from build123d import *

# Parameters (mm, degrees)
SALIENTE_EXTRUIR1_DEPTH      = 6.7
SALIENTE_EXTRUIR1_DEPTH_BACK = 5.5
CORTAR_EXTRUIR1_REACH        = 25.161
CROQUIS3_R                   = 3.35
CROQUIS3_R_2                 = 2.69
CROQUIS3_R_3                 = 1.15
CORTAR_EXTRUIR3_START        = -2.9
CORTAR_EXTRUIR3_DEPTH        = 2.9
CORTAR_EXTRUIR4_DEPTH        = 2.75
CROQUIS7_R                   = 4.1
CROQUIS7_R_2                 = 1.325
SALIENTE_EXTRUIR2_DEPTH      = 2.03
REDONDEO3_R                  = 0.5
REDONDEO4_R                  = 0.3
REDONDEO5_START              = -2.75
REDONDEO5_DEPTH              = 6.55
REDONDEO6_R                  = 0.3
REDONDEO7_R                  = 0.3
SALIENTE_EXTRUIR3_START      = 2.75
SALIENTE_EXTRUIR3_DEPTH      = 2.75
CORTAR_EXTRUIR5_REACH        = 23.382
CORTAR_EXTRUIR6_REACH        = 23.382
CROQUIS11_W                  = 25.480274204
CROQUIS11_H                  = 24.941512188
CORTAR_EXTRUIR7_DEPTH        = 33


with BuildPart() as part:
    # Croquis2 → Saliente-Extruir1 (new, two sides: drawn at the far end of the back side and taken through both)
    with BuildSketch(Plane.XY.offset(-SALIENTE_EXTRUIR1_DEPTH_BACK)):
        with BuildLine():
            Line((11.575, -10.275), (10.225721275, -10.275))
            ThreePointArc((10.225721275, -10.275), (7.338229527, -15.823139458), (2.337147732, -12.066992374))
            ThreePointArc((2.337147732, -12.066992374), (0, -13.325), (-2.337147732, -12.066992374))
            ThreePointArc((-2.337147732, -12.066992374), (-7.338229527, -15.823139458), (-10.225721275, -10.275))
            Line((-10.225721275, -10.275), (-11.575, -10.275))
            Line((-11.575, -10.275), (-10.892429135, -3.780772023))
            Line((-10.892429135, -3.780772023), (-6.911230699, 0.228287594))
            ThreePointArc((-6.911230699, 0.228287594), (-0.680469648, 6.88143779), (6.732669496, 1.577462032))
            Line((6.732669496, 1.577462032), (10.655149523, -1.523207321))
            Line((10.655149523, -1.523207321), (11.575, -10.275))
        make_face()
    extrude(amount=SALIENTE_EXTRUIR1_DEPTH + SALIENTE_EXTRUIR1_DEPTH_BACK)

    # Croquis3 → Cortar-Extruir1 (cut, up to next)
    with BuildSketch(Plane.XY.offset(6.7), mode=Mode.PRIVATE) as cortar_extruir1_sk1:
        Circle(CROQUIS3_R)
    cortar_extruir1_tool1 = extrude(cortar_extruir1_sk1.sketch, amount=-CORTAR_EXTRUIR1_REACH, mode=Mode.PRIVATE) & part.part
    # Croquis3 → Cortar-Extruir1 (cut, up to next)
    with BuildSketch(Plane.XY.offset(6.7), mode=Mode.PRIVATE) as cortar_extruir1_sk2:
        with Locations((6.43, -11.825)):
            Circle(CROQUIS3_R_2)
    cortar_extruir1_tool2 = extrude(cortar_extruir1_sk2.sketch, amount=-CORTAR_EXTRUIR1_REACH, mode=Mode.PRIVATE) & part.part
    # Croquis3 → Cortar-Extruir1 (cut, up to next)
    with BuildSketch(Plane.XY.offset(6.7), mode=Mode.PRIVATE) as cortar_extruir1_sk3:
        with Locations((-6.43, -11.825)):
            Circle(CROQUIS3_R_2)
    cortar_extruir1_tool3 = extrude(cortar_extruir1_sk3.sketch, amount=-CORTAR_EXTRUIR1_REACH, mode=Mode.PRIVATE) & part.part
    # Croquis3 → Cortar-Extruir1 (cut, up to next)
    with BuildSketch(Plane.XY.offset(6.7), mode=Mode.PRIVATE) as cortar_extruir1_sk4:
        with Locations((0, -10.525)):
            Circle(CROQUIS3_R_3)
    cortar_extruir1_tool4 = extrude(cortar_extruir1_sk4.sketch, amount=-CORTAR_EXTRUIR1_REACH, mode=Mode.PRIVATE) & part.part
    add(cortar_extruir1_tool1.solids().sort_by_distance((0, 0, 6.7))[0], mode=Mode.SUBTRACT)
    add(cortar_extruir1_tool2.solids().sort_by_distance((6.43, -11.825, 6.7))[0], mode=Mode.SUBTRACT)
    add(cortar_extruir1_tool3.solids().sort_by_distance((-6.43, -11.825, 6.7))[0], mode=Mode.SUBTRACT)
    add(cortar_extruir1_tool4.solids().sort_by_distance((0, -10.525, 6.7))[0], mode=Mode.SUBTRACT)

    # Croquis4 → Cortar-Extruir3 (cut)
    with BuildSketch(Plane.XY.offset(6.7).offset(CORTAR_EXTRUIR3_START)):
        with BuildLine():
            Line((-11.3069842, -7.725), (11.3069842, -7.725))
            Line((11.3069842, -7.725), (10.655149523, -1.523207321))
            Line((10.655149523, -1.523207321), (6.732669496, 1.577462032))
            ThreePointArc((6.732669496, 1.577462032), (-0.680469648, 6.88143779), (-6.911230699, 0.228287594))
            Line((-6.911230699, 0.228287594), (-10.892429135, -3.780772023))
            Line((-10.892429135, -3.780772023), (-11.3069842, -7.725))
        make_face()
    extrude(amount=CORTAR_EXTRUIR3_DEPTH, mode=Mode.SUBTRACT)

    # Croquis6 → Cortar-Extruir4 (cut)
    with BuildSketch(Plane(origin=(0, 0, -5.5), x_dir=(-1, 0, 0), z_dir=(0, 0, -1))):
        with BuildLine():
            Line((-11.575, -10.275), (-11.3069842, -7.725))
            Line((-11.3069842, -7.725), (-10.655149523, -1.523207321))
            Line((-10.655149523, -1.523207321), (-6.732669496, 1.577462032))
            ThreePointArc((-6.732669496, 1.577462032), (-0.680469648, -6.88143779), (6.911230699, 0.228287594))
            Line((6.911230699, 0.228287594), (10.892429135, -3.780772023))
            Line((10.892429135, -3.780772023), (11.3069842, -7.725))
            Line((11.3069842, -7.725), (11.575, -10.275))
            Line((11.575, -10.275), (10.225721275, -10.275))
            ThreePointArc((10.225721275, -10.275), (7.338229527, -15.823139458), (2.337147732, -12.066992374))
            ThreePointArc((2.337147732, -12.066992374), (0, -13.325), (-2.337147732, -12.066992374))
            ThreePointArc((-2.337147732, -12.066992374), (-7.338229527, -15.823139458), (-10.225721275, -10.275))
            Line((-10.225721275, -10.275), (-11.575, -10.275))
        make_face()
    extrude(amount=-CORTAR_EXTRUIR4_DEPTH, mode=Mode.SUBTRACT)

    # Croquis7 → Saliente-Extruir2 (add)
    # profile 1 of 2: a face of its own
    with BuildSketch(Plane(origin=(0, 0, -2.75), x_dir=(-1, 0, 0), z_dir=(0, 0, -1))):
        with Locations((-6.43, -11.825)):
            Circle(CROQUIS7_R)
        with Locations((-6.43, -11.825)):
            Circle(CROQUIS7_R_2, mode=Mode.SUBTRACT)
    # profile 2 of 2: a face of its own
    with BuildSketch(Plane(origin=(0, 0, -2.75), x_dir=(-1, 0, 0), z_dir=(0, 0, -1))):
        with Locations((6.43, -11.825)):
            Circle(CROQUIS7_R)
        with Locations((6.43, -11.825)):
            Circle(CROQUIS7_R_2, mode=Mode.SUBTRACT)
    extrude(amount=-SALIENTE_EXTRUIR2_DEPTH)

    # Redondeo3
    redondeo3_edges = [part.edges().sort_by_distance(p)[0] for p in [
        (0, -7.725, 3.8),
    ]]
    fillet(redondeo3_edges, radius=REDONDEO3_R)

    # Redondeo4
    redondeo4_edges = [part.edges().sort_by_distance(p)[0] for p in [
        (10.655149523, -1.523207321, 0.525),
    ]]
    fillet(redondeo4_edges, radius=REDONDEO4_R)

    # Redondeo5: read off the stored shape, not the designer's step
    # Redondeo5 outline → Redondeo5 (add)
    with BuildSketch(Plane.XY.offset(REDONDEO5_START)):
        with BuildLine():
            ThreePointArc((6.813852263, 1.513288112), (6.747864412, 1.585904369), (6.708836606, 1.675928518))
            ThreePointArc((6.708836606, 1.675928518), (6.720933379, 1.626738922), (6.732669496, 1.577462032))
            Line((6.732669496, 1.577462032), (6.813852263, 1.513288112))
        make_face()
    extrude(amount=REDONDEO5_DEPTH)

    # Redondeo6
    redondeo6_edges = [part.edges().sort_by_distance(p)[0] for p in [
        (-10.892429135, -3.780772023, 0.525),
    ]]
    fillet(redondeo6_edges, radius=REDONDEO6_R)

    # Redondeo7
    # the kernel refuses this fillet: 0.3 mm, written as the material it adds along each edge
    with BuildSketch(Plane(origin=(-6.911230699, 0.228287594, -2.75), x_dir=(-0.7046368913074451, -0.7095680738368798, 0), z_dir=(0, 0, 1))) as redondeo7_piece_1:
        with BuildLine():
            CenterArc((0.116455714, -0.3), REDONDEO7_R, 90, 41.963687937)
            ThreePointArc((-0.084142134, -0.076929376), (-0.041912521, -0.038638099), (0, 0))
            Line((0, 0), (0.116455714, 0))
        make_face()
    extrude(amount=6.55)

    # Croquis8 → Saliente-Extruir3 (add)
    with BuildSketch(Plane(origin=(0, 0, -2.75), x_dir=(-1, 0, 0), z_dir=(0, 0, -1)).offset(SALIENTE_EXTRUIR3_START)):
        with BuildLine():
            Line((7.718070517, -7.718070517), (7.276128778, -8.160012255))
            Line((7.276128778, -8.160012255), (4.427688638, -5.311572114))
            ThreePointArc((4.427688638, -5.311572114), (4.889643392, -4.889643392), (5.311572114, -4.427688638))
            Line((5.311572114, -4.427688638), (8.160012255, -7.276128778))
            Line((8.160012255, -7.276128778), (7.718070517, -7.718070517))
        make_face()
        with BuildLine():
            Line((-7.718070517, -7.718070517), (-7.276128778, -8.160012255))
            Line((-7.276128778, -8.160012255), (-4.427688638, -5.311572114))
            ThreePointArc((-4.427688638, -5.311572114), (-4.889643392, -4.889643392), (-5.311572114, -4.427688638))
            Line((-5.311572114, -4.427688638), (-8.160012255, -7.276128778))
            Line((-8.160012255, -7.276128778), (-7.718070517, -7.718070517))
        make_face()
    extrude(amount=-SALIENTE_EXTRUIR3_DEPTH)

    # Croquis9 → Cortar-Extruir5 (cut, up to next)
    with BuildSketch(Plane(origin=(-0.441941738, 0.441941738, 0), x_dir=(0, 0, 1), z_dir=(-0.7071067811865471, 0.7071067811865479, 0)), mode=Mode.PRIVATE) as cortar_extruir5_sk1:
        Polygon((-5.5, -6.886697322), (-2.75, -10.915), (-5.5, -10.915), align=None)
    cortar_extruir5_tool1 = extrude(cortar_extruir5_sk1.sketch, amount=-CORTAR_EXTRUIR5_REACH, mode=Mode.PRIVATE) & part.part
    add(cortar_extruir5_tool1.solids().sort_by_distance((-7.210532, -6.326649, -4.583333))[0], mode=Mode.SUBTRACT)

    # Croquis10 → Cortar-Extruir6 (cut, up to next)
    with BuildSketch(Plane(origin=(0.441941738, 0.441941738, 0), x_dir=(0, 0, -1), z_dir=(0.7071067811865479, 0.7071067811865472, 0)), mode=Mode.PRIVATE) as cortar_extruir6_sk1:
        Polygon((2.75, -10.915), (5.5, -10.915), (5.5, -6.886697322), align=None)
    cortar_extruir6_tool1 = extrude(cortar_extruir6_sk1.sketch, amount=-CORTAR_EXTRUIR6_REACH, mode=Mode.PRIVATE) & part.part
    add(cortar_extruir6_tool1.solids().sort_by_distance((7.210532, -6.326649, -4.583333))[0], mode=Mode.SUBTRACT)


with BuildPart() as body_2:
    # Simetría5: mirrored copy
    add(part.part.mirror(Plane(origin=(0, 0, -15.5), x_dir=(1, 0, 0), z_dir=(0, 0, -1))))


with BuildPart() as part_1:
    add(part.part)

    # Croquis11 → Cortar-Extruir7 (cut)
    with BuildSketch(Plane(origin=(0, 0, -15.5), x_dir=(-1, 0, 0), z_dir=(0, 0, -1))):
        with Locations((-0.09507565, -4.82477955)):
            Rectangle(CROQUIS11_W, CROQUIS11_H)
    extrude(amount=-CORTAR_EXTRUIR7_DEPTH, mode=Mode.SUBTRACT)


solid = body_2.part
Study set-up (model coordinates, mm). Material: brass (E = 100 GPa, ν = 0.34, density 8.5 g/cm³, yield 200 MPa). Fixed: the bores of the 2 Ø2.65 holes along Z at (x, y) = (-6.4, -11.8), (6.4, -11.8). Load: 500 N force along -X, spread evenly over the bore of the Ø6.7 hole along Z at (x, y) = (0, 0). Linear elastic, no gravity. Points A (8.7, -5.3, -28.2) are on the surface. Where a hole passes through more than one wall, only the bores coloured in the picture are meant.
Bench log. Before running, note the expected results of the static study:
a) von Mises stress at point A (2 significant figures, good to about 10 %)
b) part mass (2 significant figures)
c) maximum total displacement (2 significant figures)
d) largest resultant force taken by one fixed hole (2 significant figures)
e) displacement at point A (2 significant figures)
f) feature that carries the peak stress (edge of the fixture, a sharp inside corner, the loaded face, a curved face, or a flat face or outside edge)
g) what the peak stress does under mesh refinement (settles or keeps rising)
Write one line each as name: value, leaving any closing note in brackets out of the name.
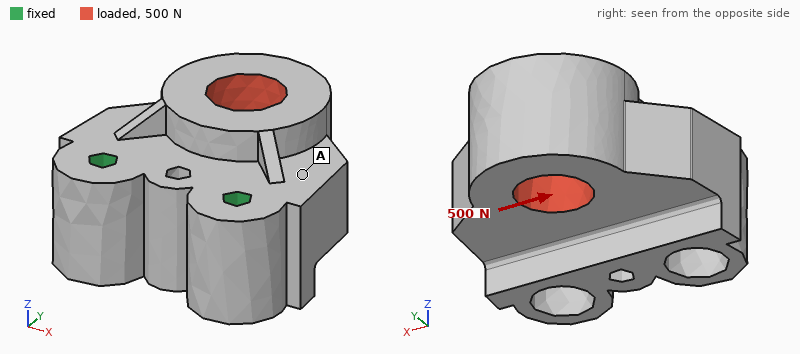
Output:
von Mises stress at point A: 9.4 MPa
part mass: 23 g
maximum total displacement: 6.5 µm
largest resultant force taken by one fixed hole: 470 N
displacement at point A: 3.0 µm
feature that carries the peak stress: edge of the fixture
what the peak stress does under mesh refinement: keeps rising
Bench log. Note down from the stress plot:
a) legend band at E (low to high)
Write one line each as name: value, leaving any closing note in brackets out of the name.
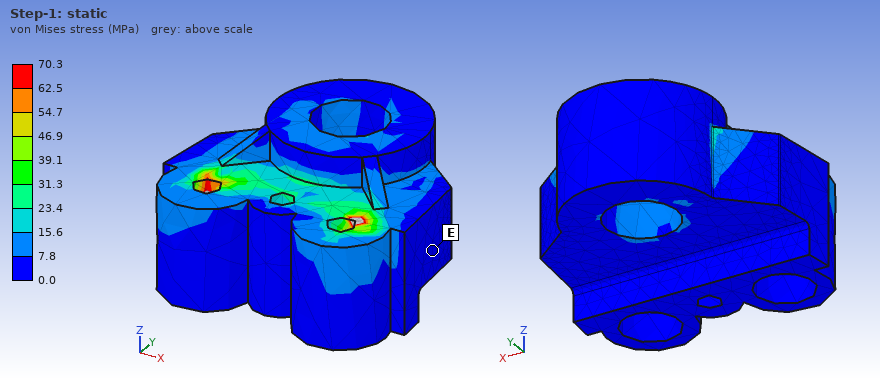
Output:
legend band at E: 0.0 to 7.8 MPa
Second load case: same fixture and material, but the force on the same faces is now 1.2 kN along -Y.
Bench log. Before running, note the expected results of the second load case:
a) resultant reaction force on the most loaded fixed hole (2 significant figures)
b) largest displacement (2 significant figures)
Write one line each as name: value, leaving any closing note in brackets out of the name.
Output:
resultant reaction force on the most loaded fixed hole: 610 N
largest displacement: 9.1 µm
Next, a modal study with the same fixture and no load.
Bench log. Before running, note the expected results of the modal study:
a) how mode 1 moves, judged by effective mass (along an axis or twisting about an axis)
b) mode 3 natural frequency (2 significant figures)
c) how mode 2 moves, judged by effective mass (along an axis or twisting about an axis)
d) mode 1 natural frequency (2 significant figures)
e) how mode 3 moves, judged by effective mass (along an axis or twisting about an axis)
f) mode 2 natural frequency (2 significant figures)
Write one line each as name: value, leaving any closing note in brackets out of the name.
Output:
how mode 1 moves, judged by effective mass: along Z
mode 3 natural frequency: 18 kHz
how mode 2 moves, judged by effective mass: along X
mode 1 natural frequency: 4800 Hz
how mode 3 moves, judged by effective mass: along X
mode 2 natural frequency: 14 kHz
